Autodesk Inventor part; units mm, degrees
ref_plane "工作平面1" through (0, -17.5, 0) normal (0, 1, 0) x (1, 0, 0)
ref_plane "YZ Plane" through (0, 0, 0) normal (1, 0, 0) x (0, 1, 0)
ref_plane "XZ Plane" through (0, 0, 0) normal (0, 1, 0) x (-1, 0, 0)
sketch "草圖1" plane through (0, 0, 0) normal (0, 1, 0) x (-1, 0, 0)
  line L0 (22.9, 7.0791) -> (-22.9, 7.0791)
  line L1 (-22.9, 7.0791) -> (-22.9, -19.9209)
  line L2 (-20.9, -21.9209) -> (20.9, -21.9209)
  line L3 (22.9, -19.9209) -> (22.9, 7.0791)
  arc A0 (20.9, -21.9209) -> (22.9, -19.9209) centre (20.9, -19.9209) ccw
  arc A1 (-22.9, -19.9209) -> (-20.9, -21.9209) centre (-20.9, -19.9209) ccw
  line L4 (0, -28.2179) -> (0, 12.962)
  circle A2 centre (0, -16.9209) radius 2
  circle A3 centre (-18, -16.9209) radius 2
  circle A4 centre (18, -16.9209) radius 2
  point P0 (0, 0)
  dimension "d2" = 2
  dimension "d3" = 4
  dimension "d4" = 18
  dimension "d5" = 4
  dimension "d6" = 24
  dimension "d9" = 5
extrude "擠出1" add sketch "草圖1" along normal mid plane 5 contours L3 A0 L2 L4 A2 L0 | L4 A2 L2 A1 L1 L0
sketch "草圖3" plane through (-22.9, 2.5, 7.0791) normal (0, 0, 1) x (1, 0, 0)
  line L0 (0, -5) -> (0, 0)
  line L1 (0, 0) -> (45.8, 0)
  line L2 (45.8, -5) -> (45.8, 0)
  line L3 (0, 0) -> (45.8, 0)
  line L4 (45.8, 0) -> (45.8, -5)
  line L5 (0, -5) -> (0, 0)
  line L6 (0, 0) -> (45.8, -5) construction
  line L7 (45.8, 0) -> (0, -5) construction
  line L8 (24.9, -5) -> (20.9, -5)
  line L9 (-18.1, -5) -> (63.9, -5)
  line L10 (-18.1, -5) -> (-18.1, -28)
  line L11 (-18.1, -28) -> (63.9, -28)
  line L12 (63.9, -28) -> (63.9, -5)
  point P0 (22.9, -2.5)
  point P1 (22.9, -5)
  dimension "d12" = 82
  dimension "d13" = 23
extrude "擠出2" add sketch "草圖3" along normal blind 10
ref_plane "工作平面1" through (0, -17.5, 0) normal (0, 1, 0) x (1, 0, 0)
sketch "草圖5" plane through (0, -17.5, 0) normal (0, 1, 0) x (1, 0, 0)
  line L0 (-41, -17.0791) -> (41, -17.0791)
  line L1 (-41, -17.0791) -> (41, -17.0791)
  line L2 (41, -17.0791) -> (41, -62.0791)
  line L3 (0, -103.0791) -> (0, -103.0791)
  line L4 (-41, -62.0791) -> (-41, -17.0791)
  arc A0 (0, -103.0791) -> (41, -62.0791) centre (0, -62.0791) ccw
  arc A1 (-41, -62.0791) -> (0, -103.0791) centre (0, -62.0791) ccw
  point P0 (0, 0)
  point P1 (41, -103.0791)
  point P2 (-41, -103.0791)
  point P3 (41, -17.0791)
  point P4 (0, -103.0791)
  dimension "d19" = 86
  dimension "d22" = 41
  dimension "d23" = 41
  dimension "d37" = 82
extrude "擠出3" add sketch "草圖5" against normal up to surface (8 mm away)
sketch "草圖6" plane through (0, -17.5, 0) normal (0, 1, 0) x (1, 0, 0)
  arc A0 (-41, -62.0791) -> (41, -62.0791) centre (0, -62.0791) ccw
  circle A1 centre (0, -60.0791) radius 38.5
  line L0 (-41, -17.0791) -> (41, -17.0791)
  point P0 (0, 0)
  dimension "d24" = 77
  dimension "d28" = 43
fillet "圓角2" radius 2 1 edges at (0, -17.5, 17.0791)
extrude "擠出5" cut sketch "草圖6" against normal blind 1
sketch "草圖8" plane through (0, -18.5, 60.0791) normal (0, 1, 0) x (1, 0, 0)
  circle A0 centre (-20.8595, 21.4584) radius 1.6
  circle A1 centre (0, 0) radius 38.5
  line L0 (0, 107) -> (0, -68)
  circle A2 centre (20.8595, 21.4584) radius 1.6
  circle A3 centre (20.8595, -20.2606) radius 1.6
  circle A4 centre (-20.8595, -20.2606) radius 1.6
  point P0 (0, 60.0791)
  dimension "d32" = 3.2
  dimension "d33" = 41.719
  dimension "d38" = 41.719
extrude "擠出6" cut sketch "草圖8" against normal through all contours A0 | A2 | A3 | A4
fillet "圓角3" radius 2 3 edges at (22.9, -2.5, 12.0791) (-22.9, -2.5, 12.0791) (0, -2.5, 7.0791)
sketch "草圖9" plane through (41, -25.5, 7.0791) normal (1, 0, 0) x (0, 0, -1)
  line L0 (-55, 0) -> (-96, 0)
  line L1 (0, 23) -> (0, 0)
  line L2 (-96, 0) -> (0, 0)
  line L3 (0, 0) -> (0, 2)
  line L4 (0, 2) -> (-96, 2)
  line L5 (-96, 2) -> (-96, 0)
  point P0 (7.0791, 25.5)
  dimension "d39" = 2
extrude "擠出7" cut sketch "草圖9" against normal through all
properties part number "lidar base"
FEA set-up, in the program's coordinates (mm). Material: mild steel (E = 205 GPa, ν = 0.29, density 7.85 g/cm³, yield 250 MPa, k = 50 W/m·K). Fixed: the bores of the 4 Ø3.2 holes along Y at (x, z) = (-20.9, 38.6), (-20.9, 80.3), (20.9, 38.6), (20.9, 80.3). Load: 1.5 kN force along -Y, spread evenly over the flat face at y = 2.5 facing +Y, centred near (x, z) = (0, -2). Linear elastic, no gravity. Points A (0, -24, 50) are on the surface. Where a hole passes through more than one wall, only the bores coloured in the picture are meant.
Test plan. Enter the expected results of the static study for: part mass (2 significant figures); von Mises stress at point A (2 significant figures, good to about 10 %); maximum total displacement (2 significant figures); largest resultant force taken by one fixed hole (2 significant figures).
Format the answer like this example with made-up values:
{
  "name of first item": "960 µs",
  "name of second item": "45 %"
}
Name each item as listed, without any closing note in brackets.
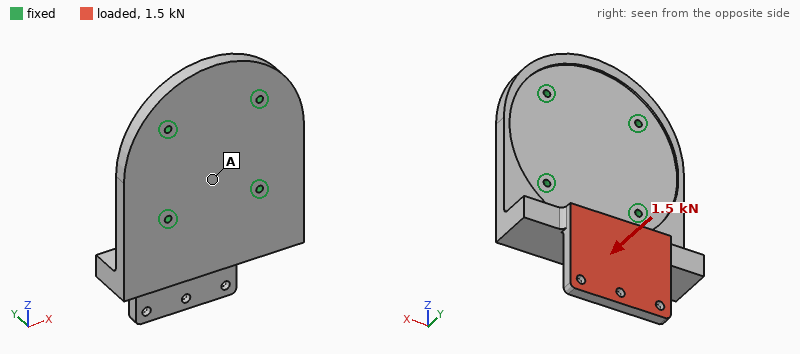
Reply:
{
  "part mass": "470 g",
  "von Mises stress at point A": "37 MPa",
  "maximum total displacement": "0.37 mm",
  "largest resultant force taken by one fixed hole": "1.1 kN"
}
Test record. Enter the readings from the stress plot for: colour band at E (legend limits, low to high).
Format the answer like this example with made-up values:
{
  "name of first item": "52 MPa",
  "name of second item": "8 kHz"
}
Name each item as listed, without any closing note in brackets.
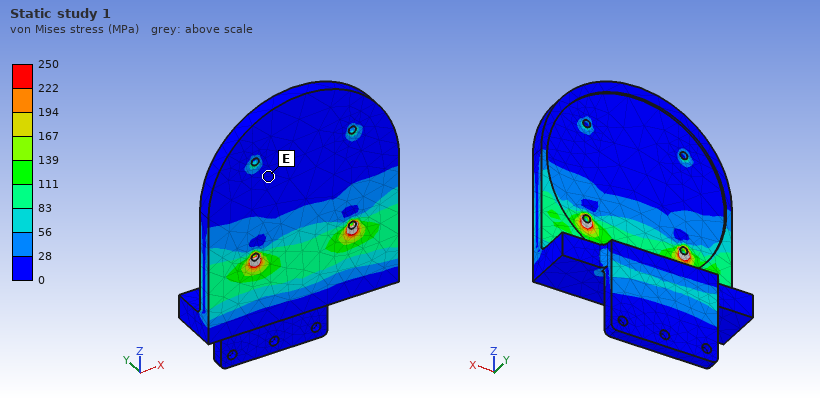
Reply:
{
  "colour band at E": "0 to 28 MPa"
}
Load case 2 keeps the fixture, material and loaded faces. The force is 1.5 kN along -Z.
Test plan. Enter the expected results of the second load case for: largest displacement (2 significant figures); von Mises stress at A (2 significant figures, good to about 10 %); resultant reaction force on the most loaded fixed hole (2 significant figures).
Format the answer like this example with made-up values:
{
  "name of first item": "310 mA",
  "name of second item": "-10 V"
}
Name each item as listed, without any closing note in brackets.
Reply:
{
  "largest displacement": "0.25 mm",
  "von Mises stress at A": "19 MPa",
  "resultant reaction force on the most loaded fixed hole": "630 N"
}
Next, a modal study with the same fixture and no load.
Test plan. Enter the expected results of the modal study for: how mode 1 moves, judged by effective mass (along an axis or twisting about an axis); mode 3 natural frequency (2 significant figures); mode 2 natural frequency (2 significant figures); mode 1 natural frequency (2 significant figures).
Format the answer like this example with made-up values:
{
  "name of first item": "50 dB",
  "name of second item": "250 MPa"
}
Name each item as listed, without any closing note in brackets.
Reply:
{
  "how mode 1 moves, judged by effective mass": "along Y",
  "mode 3 natural frequency": "4900 Hz",
  "mode 2 natural frequency": "2900 Hz",
  "mode 1 natural frequency": "1100 Hz"
}
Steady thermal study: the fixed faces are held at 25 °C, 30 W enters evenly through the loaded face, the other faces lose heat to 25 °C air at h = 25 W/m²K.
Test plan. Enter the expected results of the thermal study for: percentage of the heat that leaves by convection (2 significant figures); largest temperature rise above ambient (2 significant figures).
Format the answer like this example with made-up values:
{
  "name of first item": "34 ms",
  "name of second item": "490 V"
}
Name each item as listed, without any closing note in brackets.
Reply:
{
  "percentage of the heat that leaves by convection": "33 %",
  "largest temperature rise above ambient": "74 K"
}
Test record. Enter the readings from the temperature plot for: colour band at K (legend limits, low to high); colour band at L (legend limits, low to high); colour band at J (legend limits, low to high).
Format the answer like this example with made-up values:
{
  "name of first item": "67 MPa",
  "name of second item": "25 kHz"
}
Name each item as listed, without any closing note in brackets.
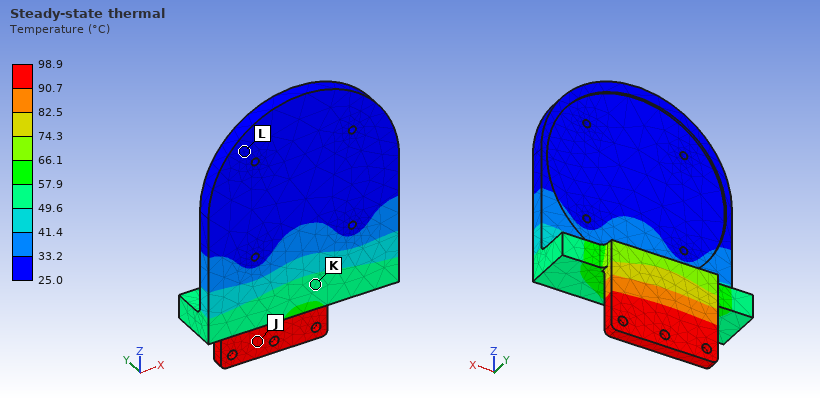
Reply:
{
  "colour band at K": "49.6 to 57.9 °C",
  "colour band at L": "25.0 to 33.2 °C",
  "colour band at J": "90.7 to 98.9 °C"
}
